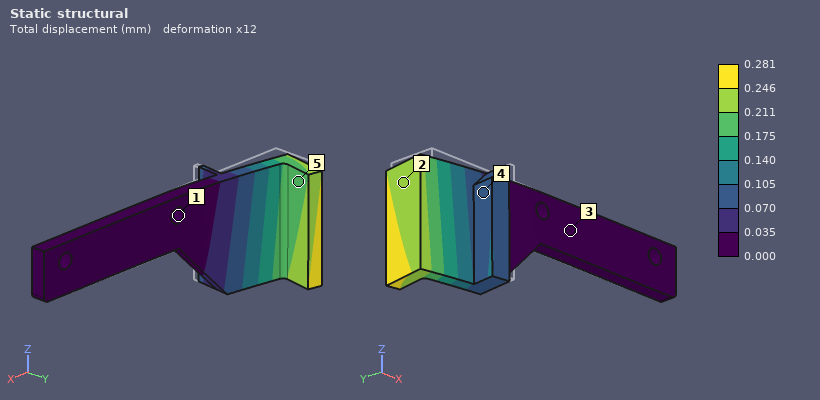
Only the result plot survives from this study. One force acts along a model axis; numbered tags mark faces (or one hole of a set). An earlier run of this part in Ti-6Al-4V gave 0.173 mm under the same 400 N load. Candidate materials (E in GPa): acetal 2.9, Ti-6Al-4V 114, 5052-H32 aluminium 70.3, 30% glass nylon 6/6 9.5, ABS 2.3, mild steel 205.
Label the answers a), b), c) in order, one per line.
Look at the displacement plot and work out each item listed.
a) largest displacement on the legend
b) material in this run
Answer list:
a) 0.281 mm
b) 5052-H32 aluminium
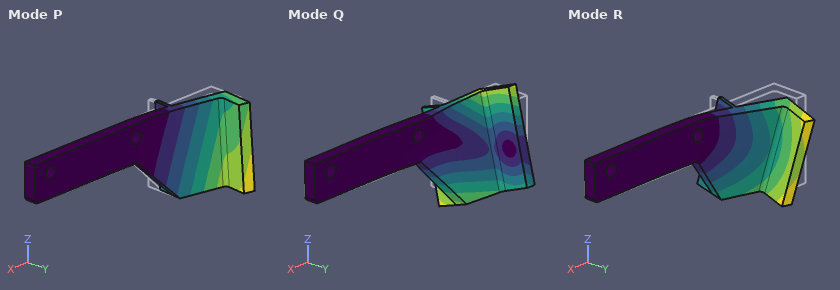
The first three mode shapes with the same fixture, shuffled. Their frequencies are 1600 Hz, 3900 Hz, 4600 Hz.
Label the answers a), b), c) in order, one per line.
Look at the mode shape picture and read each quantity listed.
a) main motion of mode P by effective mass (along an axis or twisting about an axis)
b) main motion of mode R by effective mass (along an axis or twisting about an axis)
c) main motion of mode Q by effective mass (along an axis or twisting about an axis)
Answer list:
a) along Y
b) along Z
c) along Z
